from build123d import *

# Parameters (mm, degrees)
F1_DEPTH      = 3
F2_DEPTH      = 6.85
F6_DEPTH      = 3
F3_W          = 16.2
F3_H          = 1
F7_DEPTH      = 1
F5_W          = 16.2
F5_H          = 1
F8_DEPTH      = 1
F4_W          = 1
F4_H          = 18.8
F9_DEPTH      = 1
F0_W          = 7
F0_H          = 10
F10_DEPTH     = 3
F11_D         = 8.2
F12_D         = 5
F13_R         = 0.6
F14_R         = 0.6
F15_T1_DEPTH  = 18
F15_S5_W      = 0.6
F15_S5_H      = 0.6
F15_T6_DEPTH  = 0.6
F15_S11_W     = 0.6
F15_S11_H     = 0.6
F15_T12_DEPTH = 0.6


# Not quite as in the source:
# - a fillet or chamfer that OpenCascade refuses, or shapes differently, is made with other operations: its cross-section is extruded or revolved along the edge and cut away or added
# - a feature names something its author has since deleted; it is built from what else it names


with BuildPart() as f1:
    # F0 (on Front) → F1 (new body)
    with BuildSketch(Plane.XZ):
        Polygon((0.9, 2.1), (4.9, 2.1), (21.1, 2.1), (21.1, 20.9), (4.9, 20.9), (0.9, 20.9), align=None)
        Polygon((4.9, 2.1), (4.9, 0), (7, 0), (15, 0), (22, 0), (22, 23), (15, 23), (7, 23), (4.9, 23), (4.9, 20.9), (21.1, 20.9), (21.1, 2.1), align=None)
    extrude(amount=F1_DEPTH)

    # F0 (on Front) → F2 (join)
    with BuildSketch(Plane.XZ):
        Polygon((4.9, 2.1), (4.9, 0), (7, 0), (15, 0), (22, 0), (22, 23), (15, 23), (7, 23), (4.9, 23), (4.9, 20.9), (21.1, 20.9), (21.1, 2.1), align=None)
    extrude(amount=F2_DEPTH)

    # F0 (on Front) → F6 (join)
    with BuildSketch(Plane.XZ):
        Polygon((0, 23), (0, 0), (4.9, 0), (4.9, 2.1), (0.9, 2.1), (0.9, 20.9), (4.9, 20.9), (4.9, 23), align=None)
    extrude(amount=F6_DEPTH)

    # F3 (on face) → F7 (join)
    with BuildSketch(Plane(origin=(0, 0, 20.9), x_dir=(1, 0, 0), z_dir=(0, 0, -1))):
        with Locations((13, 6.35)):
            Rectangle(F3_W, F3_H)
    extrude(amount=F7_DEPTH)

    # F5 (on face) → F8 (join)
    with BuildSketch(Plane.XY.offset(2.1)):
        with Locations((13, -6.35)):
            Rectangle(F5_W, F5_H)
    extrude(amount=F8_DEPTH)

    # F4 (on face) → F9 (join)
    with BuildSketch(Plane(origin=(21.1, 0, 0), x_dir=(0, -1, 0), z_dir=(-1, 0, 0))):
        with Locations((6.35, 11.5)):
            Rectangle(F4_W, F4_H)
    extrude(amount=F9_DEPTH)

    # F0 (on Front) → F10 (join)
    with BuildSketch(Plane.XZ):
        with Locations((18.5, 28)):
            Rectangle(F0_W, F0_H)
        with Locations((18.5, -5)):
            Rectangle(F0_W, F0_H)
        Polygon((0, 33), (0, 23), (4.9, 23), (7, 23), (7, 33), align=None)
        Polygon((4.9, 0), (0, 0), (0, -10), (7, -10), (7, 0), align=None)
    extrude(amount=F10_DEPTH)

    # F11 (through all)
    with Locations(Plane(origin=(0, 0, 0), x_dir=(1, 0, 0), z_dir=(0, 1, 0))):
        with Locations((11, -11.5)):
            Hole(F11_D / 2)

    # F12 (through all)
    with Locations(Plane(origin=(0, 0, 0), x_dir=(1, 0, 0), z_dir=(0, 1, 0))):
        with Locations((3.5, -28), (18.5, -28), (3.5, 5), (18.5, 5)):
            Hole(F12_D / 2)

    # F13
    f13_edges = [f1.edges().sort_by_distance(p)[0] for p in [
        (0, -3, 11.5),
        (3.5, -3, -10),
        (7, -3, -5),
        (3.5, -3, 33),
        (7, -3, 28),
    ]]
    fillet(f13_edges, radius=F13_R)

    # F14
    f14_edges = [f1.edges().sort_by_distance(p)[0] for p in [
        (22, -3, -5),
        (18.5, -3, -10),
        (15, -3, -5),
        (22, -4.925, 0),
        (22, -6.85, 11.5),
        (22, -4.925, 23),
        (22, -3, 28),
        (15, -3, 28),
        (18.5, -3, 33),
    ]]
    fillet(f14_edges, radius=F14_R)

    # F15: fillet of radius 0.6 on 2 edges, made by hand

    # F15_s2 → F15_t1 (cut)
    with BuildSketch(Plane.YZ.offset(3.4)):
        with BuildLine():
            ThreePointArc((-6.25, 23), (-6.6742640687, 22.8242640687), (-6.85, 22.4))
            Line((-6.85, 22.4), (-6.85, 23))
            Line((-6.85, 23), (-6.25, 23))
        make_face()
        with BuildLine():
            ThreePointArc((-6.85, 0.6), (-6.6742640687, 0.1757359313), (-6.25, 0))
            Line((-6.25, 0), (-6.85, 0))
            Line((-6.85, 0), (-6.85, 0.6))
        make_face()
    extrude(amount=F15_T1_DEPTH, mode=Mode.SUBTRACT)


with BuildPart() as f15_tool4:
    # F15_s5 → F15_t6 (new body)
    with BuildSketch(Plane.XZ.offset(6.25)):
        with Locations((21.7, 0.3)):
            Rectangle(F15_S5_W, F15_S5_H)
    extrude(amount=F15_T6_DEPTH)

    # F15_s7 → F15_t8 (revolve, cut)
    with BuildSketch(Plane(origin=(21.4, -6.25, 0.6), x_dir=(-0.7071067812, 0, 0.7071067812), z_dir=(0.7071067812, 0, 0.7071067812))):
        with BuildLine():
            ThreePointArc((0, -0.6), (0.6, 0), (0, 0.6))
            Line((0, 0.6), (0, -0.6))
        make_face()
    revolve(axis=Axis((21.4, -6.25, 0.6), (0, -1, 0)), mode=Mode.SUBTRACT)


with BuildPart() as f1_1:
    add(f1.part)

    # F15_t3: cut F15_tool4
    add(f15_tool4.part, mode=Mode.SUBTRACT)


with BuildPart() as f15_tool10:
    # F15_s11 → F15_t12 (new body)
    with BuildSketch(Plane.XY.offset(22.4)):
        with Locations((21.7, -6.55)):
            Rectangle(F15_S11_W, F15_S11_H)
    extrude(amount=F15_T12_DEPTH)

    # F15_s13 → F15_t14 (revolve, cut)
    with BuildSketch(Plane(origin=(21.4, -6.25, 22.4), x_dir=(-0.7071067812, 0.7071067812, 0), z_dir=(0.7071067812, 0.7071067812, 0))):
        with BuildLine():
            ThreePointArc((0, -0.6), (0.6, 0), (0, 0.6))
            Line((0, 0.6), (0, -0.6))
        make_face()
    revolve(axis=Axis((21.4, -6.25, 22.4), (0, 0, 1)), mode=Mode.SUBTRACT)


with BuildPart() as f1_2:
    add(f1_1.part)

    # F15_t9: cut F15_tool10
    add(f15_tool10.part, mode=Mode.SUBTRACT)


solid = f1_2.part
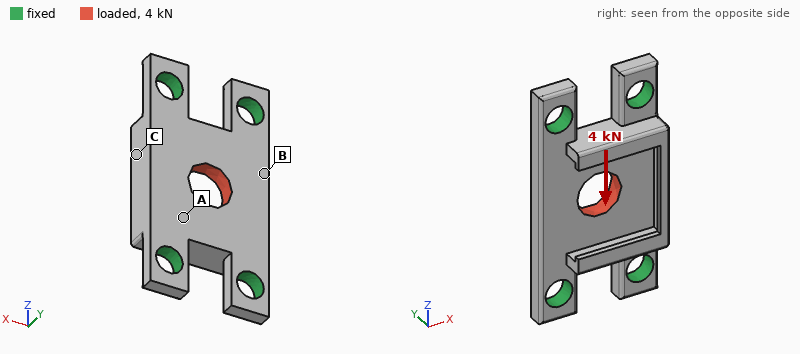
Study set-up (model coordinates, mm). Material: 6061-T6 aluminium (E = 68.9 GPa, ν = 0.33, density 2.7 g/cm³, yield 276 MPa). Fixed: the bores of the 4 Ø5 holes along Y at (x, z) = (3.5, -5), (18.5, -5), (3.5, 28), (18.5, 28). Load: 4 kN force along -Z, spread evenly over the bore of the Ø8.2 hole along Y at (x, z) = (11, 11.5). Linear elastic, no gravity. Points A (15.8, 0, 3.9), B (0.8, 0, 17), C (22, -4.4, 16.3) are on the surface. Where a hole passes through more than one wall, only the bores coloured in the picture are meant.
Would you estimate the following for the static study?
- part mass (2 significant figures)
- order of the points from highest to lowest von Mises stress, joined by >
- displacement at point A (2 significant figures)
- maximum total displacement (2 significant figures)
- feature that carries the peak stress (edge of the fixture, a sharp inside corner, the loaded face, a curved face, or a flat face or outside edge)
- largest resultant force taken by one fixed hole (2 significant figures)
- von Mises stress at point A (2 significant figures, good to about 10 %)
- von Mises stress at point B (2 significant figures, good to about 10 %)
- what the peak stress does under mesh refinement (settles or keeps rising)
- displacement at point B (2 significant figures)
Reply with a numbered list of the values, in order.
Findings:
1. 6.3 g
2. A > B > C
3. 5.5 µm
4. 10 µm
5. a sharp inside corner
6. 1.0 kN
7. 55 MPa
8. 16 MPa
9. keeps rising
10. 4.1 µm
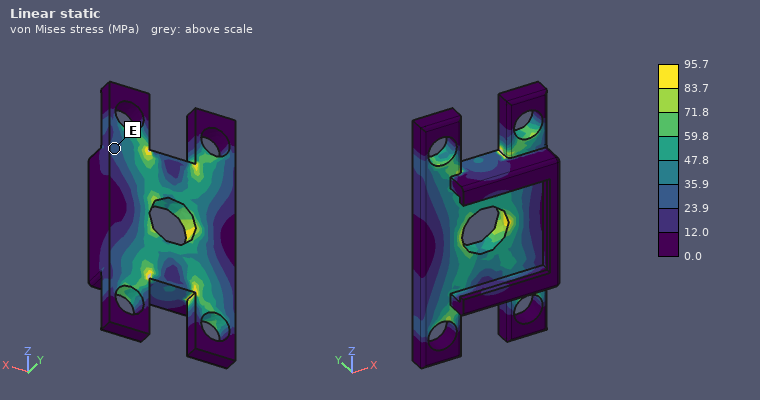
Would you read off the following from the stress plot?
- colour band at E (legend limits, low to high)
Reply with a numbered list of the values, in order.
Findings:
1. 23.9 to 35.9 MPa
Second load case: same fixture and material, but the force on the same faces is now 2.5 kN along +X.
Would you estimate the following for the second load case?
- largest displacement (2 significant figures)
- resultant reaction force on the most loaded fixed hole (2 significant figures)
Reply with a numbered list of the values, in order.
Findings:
1. 18 µm
2. 730 N
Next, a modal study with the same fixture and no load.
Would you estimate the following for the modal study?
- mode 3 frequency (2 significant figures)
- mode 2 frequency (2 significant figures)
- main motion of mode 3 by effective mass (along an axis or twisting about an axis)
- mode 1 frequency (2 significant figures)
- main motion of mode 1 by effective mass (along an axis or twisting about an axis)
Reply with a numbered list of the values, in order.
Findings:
1. 34 kHz
2. 23 kHz
3. along X
4. 17 kHz
5. along Y
